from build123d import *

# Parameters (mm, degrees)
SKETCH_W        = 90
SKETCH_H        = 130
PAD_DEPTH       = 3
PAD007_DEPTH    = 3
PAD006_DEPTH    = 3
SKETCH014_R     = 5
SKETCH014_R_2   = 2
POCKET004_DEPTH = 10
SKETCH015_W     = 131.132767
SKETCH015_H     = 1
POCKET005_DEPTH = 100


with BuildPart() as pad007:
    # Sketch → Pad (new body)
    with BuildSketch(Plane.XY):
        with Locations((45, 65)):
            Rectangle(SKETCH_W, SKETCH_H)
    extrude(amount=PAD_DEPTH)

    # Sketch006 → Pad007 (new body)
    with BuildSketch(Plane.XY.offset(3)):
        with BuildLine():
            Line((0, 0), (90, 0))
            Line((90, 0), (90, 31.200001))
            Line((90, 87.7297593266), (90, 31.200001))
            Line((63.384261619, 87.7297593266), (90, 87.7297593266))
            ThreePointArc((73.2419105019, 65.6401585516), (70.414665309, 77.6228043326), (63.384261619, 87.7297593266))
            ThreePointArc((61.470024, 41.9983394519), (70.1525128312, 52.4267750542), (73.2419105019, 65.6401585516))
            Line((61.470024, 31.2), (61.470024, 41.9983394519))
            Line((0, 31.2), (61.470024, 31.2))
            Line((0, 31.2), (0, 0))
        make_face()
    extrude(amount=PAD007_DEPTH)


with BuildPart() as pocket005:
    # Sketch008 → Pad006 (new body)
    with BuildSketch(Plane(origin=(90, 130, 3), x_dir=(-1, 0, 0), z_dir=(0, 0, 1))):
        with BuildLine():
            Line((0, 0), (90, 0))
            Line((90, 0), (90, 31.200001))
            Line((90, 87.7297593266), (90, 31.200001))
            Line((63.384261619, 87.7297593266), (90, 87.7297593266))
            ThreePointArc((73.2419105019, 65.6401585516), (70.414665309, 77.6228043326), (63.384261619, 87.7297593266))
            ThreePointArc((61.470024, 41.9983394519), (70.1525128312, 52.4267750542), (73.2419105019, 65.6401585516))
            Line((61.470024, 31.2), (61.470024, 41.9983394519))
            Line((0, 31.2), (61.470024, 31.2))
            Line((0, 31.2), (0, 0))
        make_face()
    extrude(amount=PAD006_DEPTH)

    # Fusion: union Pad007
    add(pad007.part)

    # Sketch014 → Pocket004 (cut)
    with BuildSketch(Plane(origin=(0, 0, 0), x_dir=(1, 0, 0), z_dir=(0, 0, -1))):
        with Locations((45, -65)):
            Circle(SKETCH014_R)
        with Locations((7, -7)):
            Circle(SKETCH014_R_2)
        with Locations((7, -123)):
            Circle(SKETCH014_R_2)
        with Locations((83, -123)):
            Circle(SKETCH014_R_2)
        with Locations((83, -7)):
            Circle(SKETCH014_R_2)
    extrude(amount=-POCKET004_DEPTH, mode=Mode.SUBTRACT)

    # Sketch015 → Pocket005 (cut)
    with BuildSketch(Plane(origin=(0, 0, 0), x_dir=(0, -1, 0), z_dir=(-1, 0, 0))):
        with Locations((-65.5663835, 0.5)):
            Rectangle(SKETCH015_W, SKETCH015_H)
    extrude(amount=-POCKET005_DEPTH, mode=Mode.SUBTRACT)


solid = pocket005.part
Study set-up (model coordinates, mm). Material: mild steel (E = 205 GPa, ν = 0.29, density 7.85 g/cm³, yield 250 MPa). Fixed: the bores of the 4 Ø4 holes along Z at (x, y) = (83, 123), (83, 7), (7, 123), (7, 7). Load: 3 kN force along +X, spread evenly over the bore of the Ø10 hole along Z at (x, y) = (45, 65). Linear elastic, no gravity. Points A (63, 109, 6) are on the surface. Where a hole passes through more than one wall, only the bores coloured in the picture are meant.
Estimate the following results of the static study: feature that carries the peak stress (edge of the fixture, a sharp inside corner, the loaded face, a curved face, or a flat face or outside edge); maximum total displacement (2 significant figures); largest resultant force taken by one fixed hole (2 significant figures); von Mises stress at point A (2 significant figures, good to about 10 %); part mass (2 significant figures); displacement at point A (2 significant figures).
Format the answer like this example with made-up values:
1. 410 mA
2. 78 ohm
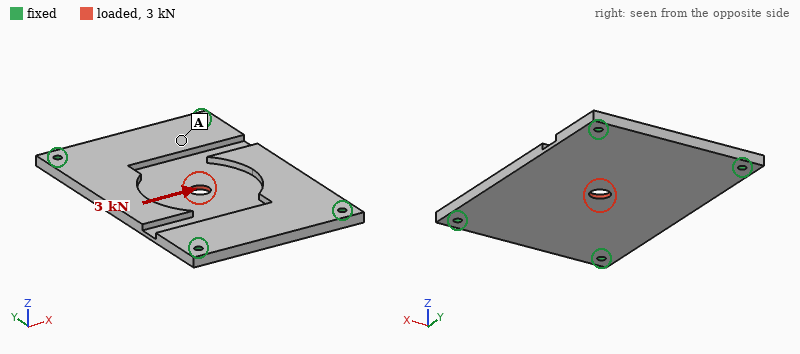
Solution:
1. the loaded face
2. 7.7 µm
3. 970 N
4. 6.6 MPa
5. 370 g
6. 1.3 µm
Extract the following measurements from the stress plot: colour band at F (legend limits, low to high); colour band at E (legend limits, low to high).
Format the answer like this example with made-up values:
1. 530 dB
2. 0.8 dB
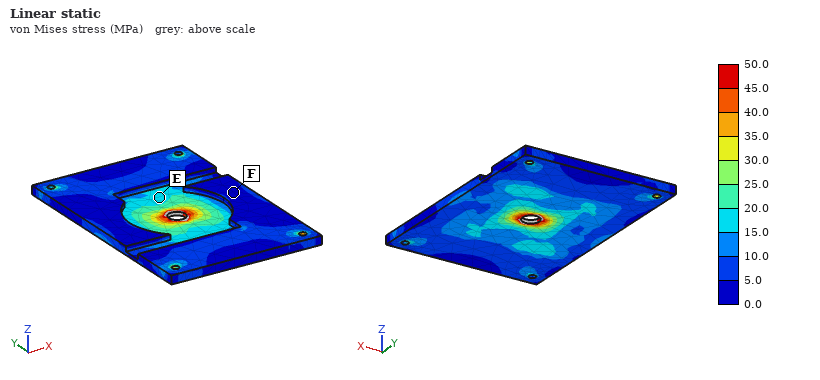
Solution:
1. 0.0 to 5.0 MPa
2. 15.0 to 20.0 MPa
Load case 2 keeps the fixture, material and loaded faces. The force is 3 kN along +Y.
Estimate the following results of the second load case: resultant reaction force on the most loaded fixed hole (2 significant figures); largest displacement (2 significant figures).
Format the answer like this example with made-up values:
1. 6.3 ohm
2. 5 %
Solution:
1. 890 N
2. 5.7 µm
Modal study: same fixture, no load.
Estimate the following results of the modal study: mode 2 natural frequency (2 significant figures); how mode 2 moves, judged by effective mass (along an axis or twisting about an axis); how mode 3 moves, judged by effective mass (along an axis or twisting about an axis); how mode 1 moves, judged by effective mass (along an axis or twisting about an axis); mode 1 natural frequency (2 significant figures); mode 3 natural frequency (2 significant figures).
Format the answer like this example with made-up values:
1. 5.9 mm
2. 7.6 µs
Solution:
1. 2200 Hz
2. twisting about Y
3. twisting about X
4. along Z
5. 1600 Hz
6. 3200 Hz
